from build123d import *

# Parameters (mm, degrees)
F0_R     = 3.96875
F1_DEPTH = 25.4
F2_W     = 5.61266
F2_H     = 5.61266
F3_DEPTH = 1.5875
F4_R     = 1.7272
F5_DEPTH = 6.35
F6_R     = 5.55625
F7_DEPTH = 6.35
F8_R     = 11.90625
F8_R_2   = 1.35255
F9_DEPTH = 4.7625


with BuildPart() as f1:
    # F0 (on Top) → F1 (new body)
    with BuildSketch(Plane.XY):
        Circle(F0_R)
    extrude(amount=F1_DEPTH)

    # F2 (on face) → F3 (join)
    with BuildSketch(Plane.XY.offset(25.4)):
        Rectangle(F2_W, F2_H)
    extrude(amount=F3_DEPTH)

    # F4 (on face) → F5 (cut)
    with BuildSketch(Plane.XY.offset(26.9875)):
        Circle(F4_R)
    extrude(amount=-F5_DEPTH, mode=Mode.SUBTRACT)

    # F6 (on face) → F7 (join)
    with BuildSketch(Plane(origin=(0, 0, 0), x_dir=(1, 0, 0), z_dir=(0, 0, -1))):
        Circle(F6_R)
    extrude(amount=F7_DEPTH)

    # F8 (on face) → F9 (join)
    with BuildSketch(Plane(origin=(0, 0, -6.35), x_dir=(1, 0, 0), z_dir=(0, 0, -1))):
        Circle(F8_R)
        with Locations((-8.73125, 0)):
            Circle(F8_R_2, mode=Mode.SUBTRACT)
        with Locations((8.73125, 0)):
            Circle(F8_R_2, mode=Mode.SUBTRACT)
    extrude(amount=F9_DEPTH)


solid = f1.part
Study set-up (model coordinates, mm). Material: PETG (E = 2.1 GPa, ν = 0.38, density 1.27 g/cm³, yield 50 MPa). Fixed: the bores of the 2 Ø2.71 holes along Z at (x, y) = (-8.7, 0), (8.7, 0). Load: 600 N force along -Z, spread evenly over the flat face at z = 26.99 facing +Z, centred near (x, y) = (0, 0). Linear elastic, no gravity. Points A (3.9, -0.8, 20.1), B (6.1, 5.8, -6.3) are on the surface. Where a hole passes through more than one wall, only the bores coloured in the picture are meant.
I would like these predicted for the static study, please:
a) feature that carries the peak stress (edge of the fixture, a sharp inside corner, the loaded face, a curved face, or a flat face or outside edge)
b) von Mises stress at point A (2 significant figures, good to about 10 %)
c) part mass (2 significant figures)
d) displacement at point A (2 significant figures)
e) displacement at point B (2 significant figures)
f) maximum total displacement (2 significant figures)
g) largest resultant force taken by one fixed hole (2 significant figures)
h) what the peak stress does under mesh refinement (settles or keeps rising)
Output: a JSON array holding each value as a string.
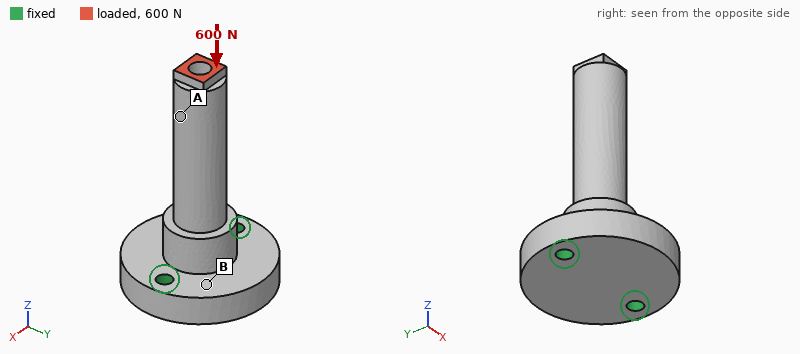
["edge of the fixture", "14 MPa", "5.0 g", "0.20 mm", "0.047 mm", "0.27 mm", "310 N", "keeps rising"]
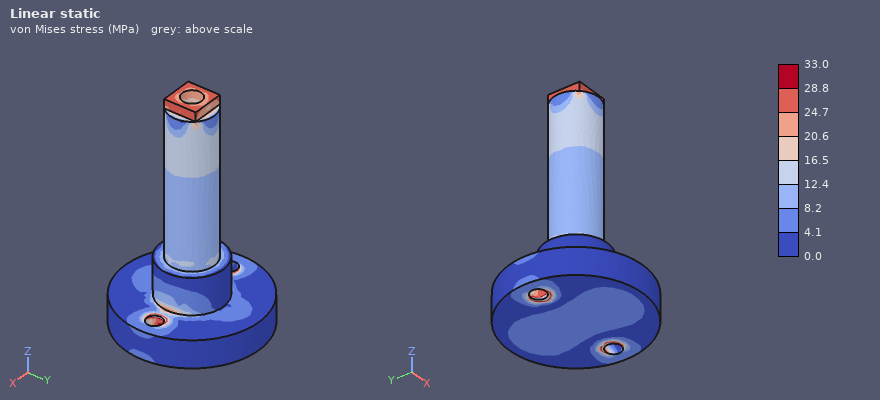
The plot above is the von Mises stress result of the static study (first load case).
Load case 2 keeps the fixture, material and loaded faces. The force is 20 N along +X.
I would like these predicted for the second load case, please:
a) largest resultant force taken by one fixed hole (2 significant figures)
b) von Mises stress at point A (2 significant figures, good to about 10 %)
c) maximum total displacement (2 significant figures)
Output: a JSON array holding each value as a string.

["48 N", "3.0 MPa", "0.50 mm"]
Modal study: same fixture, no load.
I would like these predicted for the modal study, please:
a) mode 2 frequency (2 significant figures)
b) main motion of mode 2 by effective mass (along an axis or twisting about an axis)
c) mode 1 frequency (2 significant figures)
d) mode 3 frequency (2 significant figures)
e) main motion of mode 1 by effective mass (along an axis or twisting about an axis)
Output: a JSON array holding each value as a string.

["1600 Hz", "along X", "1300 Hz", "5200 Hz", "along Y"]
